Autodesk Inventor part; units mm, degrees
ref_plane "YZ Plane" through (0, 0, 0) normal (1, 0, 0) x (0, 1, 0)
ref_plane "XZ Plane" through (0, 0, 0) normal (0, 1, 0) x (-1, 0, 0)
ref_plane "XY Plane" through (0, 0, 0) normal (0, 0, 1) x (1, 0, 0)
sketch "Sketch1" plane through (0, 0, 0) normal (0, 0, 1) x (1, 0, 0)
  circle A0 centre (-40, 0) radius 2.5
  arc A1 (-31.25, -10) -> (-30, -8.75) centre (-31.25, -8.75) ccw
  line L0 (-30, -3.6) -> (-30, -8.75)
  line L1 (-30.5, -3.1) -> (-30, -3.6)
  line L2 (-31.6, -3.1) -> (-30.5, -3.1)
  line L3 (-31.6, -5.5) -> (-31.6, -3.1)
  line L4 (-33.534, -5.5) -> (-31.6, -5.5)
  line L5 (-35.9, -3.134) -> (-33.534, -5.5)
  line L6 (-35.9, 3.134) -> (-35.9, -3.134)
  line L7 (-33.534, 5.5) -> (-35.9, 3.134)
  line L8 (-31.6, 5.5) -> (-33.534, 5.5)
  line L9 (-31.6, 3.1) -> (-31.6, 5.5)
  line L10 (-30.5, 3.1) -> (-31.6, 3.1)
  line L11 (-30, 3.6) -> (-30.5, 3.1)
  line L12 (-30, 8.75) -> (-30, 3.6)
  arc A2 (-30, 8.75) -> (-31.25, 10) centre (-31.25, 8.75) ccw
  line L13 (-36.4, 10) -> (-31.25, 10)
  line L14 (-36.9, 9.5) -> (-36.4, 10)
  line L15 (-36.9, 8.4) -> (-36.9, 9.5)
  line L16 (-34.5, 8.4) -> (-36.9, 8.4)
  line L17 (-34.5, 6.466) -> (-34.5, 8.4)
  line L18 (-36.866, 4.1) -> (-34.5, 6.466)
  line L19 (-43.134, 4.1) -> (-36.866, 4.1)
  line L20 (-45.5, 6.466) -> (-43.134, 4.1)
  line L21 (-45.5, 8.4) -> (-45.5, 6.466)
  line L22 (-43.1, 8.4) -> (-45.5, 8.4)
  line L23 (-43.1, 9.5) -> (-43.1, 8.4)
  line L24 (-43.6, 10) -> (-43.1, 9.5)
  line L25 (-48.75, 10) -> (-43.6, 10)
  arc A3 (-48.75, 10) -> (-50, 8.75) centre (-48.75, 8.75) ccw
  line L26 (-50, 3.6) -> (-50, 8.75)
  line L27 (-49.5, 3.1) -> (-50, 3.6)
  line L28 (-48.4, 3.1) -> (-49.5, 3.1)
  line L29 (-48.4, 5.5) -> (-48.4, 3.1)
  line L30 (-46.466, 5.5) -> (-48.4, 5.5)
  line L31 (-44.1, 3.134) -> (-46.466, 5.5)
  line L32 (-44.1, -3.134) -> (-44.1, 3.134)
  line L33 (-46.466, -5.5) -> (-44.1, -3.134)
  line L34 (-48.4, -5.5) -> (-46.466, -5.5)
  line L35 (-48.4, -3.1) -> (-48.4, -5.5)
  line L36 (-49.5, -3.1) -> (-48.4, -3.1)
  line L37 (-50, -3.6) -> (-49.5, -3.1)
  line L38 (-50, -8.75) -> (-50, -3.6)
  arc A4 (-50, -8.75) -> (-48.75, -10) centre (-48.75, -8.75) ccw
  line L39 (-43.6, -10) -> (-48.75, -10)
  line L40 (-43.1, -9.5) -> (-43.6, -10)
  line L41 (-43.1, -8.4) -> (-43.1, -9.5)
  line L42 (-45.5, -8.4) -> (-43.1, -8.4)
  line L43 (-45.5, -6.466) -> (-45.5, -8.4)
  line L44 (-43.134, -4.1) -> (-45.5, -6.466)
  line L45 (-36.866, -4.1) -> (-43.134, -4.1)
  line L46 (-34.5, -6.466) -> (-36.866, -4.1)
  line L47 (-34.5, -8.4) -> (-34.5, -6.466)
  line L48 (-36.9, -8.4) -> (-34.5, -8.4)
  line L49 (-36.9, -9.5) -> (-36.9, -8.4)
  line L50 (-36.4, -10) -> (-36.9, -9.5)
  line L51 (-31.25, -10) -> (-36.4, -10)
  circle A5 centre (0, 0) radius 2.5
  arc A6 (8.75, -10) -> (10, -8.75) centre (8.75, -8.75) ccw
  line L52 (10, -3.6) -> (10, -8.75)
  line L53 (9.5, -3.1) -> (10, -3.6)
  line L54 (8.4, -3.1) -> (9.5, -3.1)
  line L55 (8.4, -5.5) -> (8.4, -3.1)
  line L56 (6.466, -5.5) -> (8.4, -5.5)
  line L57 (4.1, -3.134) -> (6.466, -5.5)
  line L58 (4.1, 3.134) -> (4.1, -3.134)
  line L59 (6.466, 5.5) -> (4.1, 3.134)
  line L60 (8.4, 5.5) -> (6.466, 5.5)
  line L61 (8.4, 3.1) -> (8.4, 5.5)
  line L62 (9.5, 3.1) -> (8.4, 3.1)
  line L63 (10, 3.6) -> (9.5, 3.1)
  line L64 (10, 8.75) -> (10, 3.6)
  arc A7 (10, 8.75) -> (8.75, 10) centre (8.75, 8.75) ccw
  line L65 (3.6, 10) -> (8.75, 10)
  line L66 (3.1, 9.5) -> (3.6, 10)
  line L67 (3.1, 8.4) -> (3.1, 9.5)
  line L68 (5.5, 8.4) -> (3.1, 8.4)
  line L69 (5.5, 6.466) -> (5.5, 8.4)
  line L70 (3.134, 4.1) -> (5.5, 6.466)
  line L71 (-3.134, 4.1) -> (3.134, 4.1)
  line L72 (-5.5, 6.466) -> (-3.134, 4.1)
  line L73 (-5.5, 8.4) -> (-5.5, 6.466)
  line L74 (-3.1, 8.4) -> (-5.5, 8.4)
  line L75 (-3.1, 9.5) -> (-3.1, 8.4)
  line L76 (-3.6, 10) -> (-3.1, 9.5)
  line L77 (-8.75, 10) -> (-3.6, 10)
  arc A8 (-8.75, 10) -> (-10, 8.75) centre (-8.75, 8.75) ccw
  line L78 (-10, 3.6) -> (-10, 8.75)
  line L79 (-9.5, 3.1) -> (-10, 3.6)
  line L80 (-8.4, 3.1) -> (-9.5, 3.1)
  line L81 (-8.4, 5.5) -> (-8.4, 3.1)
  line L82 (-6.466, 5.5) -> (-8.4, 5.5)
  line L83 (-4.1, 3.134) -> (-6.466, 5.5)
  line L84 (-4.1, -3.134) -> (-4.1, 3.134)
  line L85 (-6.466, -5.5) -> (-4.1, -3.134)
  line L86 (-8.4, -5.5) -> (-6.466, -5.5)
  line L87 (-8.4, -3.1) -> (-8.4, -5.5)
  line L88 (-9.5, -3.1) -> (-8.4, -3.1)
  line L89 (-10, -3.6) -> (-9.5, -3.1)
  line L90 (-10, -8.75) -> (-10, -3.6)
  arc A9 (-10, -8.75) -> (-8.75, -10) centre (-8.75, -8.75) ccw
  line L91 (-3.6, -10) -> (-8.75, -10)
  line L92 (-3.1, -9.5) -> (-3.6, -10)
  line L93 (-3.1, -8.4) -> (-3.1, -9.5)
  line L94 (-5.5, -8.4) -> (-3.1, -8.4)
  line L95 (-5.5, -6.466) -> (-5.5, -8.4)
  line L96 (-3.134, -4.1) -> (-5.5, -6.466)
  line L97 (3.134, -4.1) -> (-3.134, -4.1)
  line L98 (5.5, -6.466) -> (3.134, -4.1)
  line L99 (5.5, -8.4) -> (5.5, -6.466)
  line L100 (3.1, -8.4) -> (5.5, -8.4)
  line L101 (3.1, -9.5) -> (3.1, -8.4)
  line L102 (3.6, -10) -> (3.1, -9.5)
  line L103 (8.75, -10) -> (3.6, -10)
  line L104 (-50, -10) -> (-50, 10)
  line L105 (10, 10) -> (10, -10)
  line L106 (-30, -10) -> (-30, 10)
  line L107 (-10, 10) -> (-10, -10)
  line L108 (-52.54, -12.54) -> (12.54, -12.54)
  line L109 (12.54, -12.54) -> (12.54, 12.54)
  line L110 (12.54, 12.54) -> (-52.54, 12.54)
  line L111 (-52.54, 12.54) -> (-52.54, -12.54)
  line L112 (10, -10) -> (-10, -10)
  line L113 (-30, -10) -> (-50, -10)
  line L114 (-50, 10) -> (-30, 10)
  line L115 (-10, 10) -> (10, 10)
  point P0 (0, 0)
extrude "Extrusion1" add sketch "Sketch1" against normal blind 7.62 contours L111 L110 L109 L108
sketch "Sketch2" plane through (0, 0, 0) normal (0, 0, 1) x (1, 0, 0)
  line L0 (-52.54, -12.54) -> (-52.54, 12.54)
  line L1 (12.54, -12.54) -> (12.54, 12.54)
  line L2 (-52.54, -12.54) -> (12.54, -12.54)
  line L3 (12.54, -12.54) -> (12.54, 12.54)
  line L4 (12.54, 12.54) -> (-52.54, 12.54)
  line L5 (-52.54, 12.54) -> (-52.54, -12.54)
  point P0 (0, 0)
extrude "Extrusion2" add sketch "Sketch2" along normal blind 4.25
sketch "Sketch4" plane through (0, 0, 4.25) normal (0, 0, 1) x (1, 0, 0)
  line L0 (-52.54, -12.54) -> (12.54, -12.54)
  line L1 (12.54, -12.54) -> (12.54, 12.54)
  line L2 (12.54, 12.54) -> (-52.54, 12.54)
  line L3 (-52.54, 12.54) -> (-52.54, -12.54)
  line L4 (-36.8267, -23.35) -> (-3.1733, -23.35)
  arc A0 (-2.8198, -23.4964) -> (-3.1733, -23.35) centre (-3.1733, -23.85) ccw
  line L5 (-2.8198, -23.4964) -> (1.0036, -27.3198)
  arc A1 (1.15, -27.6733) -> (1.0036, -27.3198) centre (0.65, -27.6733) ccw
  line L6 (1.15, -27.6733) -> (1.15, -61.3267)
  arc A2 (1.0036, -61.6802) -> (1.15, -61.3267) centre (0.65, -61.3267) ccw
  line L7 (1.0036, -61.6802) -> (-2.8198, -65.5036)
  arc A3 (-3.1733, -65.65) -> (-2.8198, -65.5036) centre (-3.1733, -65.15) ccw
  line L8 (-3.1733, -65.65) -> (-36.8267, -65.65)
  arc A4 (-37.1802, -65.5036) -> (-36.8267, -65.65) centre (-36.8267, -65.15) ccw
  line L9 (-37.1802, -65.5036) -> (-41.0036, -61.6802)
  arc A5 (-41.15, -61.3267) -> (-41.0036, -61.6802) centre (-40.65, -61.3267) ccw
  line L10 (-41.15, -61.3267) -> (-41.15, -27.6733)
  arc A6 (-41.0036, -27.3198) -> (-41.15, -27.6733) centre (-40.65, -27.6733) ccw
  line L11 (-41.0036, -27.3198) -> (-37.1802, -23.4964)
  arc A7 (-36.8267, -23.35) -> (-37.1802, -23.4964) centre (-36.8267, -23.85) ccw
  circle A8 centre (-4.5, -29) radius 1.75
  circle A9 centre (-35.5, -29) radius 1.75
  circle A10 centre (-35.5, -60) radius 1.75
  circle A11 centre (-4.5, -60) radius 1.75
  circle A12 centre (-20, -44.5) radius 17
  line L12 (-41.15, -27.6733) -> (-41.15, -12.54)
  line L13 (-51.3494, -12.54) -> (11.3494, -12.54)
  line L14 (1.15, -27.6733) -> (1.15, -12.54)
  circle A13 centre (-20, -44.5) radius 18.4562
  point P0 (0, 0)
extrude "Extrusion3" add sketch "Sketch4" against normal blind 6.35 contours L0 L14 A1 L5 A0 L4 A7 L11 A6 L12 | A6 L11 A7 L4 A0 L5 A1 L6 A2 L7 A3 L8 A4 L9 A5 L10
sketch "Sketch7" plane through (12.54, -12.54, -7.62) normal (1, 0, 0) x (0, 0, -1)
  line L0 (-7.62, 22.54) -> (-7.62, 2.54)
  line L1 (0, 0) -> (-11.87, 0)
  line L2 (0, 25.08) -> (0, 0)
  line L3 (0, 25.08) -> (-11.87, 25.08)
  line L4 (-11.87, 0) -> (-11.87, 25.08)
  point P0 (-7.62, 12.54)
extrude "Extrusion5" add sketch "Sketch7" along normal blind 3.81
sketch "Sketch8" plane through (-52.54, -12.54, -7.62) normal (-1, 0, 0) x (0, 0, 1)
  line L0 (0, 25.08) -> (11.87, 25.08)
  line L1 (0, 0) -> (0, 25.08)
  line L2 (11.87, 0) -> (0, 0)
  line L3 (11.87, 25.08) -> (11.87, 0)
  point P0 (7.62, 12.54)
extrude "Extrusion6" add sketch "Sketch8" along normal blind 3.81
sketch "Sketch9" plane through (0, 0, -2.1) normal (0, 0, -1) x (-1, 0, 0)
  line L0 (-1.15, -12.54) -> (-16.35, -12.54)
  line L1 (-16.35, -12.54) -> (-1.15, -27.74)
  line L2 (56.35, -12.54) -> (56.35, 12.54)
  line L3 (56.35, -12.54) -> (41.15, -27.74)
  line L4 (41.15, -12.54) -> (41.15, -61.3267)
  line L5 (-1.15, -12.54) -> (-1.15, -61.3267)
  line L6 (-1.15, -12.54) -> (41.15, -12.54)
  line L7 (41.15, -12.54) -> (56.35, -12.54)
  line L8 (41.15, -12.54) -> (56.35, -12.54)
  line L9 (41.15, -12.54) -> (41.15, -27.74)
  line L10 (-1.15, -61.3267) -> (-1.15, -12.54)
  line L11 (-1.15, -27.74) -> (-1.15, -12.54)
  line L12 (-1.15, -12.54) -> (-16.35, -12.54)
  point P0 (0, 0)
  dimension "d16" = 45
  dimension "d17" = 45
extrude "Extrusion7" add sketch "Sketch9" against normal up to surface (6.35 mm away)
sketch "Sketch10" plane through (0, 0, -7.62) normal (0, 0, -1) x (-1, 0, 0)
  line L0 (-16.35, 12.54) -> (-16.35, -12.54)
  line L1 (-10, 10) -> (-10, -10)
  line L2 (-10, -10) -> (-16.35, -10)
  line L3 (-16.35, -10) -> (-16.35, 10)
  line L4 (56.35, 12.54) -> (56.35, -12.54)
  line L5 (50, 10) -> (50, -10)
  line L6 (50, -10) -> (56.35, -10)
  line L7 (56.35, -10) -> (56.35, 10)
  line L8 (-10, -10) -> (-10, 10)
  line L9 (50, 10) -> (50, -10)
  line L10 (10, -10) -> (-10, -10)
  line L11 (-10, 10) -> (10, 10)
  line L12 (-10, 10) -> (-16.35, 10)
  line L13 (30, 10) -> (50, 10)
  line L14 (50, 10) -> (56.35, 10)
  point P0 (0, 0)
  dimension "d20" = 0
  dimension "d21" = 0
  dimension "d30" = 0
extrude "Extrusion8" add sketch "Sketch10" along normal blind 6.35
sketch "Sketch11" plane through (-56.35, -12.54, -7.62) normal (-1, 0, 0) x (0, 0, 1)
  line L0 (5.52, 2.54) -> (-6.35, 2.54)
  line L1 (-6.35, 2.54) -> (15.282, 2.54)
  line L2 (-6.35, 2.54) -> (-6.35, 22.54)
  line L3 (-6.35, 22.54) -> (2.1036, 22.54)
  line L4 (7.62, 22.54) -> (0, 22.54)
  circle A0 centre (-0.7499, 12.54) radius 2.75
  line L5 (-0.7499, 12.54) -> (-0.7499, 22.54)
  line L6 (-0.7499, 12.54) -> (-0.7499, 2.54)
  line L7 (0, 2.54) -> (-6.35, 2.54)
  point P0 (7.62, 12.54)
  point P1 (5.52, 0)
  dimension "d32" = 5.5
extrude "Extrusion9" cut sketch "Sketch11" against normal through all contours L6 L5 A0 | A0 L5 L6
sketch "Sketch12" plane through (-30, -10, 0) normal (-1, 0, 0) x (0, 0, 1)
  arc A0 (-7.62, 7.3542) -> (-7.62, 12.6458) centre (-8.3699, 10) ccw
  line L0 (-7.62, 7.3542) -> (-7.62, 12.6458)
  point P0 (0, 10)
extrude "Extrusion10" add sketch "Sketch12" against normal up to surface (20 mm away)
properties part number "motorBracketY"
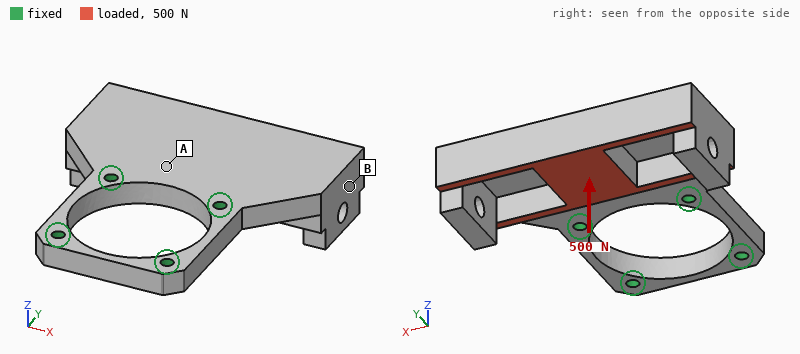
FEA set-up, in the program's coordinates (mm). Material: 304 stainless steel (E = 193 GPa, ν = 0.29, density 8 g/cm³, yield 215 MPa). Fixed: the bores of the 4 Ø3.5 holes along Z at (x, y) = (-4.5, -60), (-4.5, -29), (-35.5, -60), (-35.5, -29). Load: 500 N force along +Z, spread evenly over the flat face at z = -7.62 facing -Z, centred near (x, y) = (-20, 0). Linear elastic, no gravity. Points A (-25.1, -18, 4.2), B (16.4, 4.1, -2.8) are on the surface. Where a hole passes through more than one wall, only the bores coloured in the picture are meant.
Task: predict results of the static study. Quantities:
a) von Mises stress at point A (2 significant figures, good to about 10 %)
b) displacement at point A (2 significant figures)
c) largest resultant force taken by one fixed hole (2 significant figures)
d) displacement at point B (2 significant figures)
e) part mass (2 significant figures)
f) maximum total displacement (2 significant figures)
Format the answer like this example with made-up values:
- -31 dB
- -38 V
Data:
- 18 MPa
- 8.6 µm
- 260 N
- 35 µm
- 200 g
- 49 µm
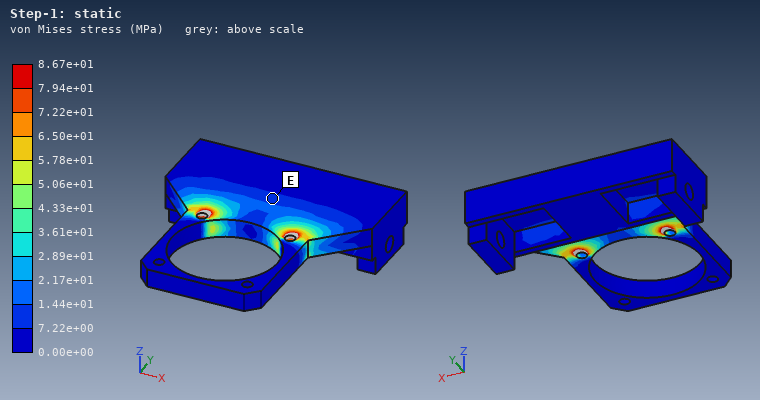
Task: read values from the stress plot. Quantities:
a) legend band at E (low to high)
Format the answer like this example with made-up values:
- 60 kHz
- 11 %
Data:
- 7.22e+00 to 1.44e+01 MPa
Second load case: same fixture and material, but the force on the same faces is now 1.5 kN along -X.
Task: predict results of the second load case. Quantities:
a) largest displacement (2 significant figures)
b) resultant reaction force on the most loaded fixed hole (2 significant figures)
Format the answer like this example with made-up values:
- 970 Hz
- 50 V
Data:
- 22 µm
- 1.5 kN
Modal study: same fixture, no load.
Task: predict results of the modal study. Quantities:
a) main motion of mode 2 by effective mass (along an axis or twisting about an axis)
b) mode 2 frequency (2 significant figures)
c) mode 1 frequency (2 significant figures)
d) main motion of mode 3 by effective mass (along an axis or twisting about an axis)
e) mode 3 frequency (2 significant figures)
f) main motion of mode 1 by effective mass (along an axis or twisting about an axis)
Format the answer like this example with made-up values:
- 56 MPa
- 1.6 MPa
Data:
- twisting about Y
- 3100 Hz
- 1600 Hz
- along X
- 6700 Hz
- along Z
